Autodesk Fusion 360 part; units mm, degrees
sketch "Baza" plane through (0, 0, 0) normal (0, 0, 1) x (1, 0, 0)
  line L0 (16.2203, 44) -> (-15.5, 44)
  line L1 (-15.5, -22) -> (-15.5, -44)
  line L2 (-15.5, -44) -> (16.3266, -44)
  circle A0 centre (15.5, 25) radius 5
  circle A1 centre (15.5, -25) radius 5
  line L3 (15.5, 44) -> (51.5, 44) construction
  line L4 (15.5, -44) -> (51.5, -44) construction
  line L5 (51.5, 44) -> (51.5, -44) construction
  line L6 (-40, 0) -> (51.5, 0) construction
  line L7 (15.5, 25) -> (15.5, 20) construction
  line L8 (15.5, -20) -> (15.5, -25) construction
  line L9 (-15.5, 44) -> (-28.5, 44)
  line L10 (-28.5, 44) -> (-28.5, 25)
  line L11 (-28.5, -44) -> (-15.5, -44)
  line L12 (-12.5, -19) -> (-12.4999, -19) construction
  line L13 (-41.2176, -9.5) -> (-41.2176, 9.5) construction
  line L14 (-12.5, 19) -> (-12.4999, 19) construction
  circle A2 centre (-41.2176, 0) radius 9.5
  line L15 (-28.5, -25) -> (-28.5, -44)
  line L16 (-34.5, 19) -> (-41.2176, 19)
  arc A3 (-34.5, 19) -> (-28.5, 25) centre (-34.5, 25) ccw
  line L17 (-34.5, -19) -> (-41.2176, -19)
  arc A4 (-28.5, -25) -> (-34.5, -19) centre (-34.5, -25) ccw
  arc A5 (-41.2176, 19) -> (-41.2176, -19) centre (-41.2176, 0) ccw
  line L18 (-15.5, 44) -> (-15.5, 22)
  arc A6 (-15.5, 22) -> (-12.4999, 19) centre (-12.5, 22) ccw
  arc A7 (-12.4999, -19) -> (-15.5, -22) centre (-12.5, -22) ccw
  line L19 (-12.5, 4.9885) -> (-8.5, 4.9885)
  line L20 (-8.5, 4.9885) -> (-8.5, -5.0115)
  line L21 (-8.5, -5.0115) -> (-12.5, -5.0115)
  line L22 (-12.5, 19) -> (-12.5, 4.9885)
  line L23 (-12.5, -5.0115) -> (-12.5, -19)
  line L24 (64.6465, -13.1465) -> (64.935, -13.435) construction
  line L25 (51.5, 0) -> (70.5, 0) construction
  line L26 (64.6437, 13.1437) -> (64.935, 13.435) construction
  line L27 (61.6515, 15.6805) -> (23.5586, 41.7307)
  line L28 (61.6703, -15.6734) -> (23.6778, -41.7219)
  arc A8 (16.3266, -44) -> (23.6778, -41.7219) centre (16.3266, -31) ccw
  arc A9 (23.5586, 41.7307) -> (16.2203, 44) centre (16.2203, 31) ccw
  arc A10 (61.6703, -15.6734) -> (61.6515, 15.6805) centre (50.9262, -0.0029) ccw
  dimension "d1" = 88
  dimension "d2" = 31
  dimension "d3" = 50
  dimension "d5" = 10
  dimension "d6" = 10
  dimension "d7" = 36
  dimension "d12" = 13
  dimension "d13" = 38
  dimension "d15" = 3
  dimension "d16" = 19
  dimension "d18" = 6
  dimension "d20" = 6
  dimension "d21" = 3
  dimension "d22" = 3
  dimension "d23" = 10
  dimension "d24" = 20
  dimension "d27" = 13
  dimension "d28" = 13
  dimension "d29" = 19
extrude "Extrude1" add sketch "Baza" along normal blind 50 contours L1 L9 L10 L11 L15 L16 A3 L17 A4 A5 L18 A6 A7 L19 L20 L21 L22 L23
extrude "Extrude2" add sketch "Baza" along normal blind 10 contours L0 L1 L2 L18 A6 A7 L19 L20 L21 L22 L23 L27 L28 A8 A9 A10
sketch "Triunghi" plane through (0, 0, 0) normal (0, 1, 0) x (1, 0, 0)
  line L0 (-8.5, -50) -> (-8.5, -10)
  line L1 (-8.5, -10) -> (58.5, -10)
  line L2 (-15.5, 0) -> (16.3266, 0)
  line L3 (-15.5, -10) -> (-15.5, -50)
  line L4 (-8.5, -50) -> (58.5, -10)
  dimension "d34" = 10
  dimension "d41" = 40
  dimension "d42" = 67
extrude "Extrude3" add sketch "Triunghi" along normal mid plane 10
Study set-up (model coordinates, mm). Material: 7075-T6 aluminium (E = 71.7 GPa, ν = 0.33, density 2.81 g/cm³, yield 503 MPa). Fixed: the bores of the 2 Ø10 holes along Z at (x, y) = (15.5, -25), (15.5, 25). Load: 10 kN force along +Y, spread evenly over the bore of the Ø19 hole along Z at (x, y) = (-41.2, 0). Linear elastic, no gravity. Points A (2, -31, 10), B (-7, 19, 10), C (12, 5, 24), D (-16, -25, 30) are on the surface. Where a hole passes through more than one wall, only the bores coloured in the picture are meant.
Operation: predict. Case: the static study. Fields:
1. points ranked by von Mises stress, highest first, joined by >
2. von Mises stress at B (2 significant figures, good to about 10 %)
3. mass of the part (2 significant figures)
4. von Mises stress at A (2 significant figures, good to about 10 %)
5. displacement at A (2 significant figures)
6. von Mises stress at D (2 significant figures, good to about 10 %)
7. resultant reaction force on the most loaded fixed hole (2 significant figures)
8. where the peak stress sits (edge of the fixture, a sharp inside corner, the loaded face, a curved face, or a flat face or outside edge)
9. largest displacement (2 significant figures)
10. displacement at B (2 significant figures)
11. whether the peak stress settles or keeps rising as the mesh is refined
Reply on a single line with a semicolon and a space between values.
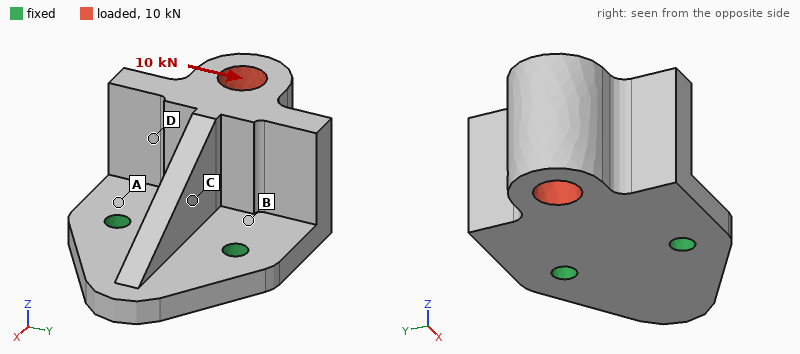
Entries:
B > A > C > D; 64 MPa; 480 g; 37 MPa; 0.023 mm; 9.9 MPa; 12 kN; edge of the fixture; 0.14 mm; 0.031 mm; keeps rising
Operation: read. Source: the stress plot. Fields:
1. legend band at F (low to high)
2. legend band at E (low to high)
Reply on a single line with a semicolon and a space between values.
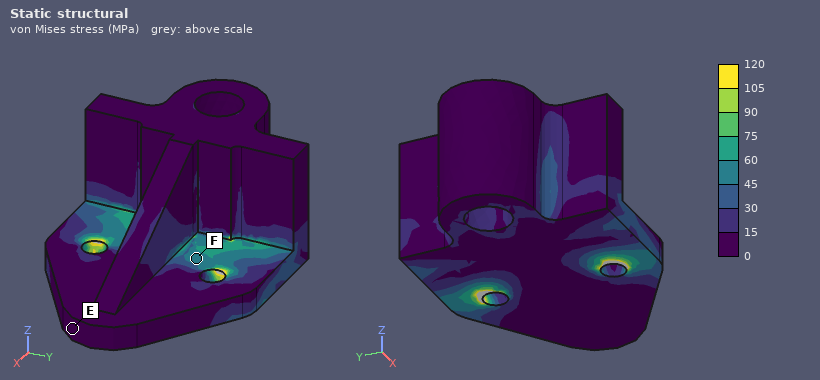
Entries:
45 to 60 MPa; 0 to 15 MPa
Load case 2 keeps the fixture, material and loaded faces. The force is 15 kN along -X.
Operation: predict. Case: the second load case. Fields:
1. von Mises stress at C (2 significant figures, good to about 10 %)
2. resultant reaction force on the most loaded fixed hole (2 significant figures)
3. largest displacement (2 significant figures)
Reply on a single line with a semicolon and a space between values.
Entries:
40 MPa; 7.5 kN; 0.43 mm
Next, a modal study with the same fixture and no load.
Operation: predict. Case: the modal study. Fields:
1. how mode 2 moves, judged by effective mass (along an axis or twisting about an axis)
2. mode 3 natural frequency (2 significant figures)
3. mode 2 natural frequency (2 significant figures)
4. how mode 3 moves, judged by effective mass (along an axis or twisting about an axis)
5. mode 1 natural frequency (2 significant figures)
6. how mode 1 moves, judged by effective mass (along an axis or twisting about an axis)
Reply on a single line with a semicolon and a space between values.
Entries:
along Y; 5500 Hz; 2700 Hz; along Z; 1400 Hz; along Z
